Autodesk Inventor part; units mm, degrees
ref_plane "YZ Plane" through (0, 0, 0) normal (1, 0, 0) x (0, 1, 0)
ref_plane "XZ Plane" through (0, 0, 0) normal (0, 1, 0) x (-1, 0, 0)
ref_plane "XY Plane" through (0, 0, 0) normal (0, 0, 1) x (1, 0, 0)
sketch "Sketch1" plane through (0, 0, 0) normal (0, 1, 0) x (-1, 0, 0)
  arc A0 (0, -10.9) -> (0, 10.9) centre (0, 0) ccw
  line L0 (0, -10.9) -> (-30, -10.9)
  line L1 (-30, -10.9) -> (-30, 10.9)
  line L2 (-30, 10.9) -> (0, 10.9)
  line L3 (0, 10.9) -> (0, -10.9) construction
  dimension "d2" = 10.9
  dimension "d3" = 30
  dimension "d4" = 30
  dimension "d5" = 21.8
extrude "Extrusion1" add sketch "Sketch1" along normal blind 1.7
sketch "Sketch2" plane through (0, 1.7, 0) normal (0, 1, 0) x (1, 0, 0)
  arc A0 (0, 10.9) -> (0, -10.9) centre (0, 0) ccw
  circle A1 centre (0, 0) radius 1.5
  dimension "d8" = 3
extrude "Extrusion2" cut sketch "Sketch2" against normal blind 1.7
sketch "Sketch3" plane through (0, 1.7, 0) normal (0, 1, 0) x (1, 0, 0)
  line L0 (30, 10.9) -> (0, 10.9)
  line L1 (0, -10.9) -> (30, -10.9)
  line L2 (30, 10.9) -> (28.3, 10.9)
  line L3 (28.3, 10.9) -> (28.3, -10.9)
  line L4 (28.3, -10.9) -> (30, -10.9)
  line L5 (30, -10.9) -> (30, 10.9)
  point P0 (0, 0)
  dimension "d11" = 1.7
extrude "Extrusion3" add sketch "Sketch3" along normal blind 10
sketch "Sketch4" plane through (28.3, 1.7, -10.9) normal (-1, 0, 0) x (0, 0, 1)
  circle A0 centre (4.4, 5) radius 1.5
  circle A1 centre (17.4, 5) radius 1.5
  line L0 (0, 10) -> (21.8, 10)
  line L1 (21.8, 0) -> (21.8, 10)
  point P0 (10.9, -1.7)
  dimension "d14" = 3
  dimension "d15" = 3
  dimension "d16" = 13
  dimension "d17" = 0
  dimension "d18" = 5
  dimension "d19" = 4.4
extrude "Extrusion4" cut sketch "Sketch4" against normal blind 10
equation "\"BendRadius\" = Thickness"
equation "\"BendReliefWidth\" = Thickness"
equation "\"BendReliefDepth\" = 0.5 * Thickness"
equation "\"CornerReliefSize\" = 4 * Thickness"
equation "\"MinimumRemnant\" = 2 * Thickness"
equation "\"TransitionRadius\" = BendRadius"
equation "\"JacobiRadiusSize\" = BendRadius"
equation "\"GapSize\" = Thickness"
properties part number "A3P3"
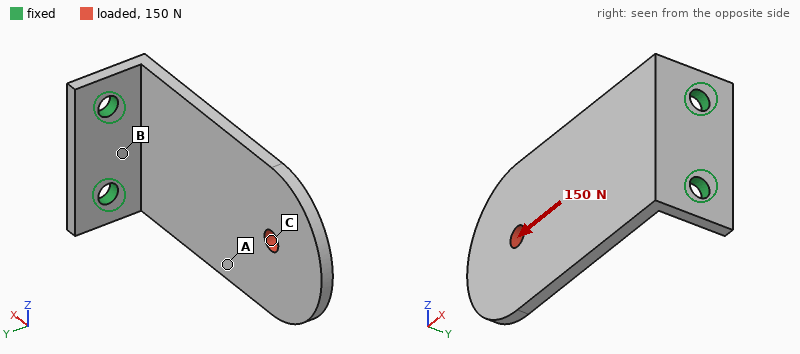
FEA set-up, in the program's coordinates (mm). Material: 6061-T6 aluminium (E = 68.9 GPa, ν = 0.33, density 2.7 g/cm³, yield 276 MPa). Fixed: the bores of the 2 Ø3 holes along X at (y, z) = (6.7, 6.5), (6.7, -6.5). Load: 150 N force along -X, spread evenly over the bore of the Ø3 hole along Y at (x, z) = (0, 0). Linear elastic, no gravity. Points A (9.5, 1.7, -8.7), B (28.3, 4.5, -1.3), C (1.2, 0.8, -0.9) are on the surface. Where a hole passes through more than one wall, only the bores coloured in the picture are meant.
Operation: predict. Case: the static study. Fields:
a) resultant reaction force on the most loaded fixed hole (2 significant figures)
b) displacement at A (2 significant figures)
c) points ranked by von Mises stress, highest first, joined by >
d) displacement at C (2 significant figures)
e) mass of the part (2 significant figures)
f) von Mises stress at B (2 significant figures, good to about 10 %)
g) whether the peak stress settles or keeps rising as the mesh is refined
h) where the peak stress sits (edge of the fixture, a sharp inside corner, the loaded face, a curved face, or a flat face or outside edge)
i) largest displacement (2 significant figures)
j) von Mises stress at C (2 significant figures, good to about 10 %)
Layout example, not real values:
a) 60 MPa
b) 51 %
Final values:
a) 75 N
b) 0.064 mm
c) B > C > A
d) 0.091 mm
e) 4.8 g
f) 27 MPa
g) keeps rising
h) edge of the fixture
i) 0.13 mm
j) 12 MPa
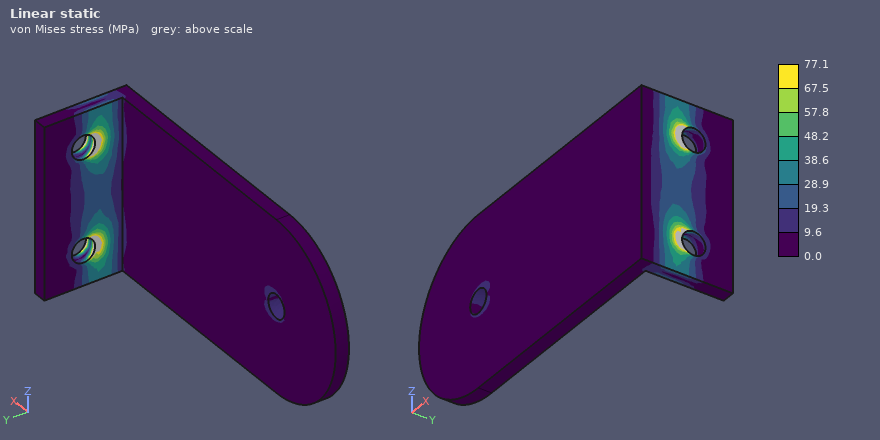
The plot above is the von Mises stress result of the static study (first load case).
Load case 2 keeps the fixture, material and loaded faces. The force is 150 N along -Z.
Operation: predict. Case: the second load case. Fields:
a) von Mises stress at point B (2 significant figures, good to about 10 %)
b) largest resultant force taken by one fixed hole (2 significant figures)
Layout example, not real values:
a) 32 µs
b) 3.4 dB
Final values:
a) 59 MPa
b) 310 N
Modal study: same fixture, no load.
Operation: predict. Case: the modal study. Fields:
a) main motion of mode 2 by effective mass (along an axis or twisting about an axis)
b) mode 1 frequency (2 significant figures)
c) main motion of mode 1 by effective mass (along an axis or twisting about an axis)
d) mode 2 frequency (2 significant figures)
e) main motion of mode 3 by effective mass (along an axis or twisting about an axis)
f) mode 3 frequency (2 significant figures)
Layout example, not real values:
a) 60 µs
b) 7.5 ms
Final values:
a) along Z
b) 820 Hz
c) along Y
d) 3100 Hz
e) along Z
f) 4100 Hz
